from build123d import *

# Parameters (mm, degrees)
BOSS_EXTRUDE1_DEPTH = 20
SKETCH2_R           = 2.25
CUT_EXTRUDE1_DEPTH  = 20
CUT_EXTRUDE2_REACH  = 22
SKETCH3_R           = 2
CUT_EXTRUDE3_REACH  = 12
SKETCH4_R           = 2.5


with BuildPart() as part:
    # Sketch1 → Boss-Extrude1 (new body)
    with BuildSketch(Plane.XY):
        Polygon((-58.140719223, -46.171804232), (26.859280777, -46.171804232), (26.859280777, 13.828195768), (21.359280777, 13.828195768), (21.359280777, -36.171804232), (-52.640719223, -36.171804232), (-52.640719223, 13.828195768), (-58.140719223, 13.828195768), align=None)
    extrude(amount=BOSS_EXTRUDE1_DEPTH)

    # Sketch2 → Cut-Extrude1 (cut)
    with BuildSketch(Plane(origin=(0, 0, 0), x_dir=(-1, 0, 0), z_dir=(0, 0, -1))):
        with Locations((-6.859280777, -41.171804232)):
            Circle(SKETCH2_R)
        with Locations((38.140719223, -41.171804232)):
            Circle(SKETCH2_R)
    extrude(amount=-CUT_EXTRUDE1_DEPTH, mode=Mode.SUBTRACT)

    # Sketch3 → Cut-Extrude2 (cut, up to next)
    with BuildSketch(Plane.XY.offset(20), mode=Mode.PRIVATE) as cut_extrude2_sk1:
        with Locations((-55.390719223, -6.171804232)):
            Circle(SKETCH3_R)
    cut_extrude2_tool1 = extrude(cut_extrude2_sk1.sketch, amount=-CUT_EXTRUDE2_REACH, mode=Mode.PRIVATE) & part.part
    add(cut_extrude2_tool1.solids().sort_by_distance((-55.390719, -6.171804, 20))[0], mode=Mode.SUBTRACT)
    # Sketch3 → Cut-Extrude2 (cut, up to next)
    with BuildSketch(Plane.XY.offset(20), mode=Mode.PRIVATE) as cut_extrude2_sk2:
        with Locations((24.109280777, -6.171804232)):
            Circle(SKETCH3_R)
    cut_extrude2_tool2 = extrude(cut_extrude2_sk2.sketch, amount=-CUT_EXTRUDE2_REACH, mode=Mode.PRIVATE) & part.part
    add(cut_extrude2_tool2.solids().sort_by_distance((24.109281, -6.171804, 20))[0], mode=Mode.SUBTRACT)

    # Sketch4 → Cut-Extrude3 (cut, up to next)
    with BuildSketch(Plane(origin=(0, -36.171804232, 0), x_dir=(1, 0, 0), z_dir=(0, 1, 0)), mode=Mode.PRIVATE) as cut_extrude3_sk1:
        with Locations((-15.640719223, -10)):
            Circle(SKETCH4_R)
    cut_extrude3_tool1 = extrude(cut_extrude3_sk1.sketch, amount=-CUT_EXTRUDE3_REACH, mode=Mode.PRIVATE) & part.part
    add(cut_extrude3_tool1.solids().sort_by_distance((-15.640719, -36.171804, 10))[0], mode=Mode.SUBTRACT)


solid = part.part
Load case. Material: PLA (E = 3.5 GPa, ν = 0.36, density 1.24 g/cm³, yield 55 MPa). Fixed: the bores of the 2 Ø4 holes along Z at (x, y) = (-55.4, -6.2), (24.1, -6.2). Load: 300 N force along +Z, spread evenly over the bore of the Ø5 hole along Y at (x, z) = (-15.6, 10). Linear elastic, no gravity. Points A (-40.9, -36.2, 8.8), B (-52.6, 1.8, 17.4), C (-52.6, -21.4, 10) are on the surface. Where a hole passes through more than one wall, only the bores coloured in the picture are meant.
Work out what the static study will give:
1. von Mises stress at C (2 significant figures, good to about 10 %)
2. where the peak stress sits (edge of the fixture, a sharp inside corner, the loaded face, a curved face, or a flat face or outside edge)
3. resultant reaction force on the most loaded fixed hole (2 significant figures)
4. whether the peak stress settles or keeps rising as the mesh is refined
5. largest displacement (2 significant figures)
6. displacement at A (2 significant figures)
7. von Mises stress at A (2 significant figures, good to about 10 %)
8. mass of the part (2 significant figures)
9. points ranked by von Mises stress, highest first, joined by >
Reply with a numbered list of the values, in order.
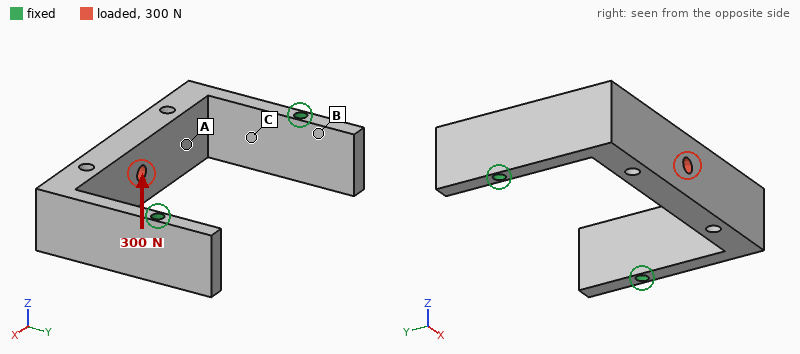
1. 6.3 MPa
2. edge of the fixture
3. 150 N
4. keeps rising
5. 0.38 mm
6. 0.23 mm
7. 3.0 MPa
8. 33 g
9. C > A > B
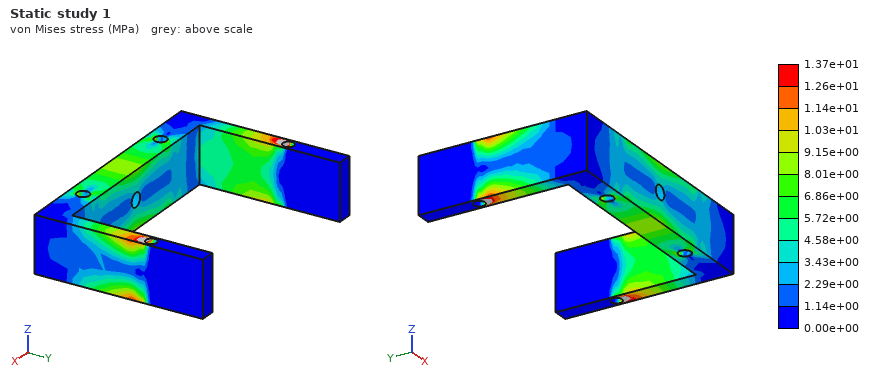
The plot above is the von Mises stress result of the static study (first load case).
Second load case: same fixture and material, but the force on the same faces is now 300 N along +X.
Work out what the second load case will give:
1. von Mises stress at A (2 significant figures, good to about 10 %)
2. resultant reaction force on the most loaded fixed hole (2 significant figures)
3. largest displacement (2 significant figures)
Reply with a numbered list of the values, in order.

1. 6.8 MPa
2. 160 N
3. 0.54 mm
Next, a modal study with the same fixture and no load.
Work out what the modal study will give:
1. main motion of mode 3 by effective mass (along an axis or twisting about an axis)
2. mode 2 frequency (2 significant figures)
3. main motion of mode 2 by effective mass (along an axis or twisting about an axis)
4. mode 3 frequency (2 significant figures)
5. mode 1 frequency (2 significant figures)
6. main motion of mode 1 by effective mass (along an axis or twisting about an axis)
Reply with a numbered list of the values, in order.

1. along Y
2. 1200 Hz
3. along Z
4. 1500 Hz
5. 820 Hz
6. along X
